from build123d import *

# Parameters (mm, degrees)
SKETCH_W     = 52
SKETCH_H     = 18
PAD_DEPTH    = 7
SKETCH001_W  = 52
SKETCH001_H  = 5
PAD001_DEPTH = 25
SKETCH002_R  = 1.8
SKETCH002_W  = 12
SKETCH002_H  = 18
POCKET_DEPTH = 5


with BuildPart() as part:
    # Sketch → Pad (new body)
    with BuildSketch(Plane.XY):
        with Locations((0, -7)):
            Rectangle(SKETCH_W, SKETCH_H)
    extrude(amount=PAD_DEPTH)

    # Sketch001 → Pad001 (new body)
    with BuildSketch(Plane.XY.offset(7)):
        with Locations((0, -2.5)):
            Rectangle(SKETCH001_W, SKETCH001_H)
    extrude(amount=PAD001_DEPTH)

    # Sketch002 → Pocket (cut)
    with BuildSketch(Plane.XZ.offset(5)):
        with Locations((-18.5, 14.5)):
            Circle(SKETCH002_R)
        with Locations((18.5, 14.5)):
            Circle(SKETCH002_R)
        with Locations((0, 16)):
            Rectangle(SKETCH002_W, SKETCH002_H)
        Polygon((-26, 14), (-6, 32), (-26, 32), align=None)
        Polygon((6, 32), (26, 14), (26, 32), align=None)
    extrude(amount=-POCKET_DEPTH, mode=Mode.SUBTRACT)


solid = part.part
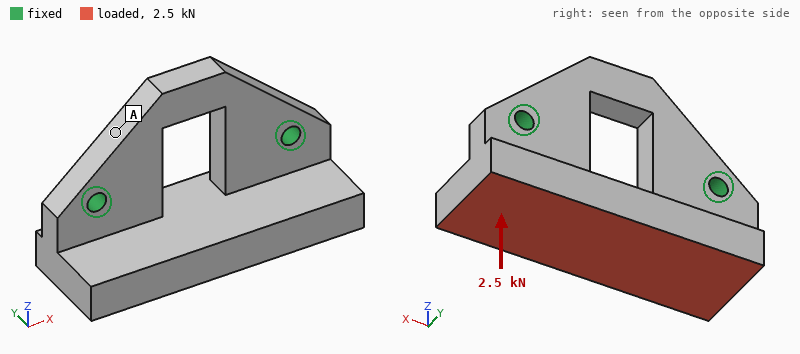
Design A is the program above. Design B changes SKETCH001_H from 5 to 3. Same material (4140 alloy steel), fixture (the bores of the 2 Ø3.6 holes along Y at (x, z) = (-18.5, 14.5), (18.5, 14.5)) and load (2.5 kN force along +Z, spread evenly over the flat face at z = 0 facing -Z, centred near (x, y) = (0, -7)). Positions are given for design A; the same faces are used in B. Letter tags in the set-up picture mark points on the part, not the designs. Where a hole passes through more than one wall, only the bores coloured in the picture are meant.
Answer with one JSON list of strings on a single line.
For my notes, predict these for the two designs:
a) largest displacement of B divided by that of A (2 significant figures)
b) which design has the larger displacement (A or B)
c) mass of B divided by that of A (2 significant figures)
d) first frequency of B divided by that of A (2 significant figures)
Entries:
["3.6", "B", "0.86", "0.52"]
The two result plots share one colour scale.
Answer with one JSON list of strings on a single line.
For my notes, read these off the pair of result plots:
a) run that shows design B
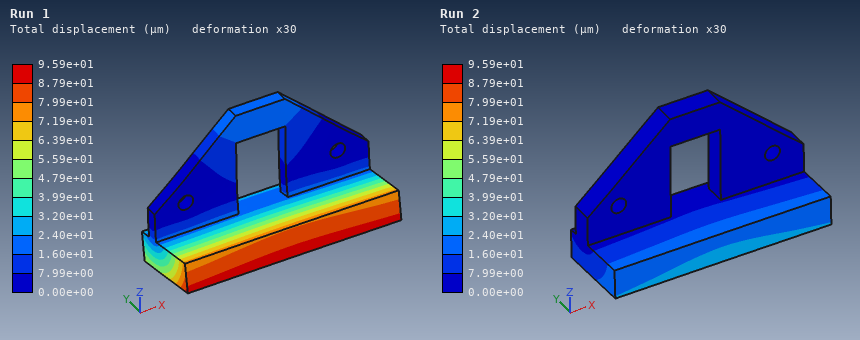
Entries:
["Run 1"]
